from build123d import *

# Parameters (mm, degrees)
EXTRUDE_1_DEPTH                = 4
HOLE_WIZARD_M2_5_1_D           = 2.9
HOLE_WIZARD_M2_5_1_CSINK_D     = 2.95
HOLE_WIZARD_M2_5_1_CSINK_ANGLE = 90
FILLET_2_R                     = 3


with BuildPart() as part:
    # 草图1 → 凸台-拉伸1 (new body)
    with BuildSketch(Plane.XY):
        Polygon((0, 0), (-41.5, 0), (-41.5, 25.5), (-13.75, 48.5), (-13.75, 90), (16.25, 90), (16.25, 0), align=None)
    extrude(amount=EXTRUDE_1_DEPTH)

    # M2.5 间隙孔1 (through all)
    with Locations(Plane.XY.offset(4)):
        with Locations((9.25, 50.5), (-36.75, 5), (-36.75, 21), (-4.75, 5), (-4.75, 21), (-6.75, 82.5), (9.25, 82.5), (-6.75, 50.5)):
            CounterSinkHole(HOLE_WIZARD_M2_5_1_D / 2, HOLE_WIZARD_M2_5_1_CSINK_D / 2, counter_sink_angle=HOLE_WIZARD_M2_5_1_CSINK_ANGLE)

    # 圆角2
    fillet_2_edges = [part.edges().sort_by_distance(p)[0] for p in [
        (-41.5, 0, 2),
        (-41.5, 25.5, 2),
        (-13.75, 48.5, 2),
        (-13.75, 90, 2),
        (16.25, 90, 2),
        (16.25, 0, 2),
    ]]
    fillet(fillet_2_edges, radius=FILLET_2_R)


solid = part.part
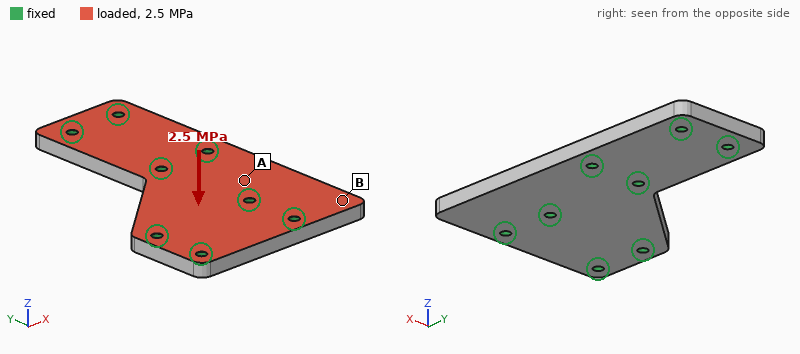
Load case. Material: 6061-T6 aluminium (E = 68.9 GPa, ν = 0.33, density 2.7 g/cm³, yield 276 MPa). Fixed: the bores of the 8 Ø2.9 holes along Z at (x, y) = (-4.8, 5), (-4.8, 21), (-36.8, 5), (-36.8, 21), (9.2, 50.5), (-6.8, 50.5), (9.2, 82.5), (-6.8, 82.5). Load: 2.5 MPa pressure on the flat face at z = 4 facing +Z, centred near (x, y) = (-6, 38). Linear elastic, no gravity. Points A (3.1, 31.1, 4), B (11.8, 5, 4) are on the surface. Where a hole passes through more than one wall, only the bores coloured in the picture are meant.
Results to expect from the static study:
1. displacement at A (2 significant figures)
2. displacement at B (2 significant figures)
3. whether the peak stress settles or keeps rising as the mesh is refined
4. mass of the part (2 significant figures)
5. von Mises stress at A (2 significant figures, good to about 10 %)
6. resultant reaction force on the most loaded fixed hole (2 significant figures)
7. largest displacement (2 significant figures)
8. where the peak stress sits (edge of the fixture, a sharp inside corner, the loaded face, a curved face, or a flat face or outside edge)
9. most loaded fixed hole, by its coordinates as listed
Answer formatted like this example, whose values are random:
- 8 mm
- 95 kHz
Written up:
- 0.036 mm
- 0.11 mm
- keeps rising
- 40 g
- 68 MPa
- 2.0 kN
- 0.14 mm
- edge of the fixture
- (-4.8, 21)
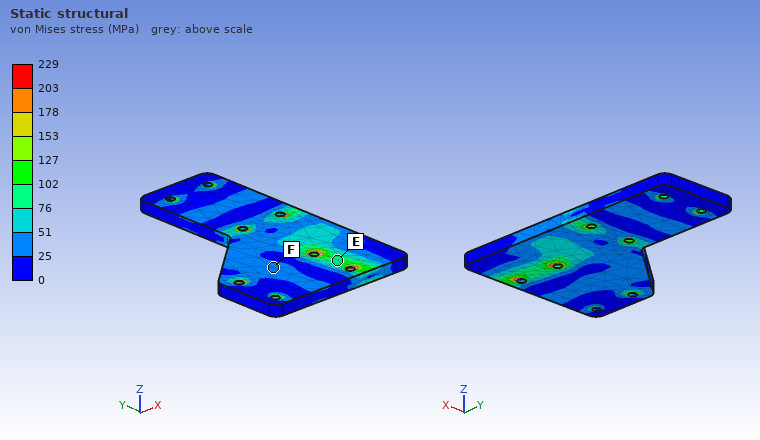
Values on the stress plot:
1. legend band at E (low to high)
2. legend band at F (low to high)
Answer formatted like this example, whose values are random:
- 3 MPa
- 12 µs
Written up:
- 76 to 102 MPa
- 25 to 51 MPa
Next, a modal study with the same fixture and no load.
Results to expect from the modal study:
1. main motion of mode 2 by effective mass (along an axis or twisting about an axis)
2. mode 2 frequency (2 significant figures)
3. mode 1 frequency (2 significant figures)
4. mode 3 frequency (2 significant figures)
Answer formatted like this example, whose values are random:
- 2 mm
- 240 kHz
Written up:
- along Z
- 13 kHz
- 8100 Hz
- 14 kHz
